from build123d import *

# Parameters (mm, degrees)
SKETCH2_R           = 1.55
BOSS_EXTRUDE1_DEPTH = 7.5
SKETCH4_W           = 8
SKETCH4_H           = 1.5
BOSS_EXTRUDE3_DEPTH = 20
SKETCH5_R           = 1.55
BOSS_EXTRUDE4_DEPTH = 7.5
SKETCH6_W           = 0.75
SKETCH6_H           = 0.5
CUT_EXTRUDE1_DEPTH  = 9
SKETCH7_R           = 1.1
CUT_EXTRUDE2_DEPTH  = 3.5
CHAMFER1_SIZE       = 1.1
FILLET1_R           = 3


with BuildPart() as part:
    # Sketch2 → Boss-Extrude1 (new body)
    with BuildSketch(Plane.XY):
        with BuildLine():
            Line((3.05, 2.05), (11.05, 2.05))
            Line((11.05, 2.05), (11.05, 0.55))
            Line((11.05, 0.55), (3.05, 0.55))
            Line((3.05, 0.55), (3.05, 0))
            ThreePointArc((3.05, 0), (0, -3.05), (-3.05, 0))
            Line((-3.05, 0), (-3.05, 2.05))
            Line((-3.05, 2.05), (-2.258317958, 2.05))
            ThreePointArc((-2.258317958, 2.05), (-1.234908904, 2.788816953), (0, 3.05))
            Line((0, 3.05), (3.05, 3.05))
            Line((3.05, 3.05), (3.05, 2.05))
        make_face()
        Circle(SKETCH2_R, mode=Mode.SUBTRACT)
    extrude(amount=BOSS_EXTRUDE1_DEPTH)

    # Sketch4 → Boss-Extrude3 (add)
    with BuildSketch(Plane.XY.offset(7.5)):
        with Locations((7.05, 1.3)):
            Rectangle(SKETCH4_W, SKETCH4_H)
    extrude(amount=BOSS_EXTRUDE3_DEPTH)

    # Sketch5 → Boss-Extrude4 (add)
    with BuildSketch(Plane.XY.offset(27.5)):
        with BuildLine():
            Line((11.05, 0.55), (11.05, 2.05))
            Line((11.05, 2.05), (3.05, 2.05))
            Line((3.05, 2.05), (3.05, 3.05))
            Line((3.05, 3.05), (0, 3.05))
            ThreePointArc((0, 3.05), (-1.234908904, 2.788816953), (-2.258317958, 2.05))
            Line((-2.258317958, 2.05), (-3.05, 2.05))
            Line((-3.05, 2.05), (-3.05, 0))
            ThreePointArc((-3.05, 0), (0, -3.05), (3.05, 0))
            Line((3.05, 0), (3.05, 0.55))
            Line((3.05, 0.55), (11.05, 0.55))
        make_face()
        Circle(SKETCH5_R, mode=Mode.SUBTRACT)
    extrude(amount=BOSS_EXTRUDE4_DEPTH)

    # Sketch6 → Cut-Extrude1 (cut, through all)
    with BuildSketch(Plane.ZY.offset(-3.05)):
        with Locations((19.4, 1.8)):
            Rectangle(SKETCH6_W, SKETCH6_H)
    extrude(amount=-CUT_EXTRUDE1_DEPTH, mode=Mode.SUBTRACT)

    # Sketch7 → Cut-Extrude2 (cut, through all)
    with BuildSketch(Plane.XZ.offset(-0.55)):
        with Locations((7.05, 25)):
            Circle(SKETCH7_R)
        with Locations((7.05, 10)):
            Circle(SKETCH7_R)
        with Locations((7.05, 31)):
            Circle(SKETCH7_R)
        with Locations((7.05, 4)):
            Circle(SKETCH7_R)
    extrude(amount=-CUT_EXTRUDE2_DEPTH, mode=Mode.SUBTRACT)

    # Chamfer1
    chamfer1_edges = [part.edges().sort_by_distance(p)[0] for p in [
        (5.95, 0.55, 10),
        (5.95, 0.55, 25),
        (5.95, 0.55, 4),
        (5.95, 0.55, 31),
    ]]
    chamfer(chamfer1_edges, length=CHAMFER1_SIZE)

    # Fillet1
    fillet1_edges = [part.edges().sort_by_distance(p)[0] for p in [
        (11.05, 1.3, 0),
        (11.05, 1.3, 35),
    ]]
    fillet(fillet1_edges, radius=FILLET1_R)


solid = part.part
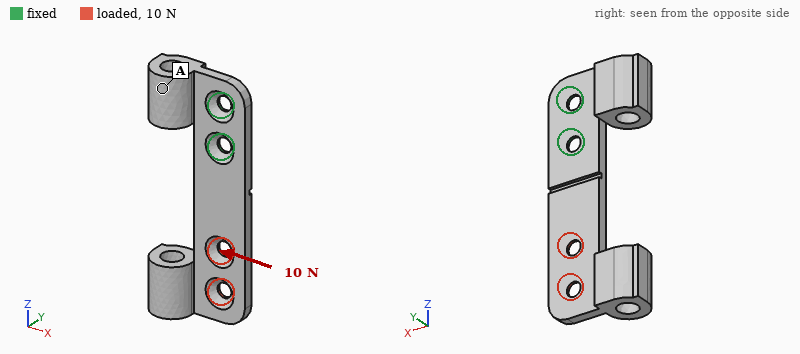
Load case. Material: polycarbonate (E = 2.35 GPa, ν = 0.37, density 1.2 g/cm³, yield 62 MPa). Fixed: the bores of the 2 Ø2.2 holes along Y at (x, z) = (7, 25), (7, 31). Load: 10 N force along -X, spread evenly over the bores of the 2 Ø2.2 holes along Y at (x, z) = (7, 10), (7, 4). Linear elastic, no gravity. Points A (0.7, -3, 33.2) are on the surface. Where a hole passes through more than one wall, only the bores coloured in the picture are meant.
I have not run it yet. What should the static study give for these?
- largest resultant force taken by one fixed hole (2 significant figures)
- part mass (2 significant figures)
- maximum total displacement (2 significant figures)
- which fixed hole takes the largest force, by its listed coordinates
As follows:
30 N
0.87 g
0.46 mm
(7, 25)
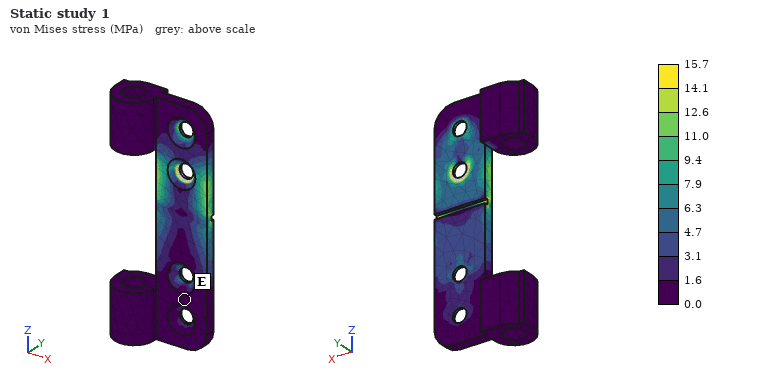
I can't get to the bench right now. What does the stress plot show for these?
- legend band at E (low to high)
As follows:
0.0 to 1.6 MPa
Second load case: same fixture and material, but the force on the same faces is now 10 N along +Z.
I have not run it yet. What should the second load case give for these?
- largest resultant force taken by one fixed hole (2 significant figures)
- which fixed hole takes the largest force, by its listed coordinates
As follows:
8.5 N
(7, 25)
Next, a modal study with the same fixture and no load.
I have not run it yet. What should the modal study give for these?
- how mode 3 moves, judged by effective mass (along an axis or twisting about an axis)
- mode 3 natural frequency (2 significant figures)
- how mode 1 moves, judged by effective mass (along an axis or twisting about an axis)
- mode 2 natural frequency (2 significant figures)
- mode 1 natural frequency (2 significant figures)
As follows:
along X
1300 Hz
along Y
1000 Hz
280 Hz
